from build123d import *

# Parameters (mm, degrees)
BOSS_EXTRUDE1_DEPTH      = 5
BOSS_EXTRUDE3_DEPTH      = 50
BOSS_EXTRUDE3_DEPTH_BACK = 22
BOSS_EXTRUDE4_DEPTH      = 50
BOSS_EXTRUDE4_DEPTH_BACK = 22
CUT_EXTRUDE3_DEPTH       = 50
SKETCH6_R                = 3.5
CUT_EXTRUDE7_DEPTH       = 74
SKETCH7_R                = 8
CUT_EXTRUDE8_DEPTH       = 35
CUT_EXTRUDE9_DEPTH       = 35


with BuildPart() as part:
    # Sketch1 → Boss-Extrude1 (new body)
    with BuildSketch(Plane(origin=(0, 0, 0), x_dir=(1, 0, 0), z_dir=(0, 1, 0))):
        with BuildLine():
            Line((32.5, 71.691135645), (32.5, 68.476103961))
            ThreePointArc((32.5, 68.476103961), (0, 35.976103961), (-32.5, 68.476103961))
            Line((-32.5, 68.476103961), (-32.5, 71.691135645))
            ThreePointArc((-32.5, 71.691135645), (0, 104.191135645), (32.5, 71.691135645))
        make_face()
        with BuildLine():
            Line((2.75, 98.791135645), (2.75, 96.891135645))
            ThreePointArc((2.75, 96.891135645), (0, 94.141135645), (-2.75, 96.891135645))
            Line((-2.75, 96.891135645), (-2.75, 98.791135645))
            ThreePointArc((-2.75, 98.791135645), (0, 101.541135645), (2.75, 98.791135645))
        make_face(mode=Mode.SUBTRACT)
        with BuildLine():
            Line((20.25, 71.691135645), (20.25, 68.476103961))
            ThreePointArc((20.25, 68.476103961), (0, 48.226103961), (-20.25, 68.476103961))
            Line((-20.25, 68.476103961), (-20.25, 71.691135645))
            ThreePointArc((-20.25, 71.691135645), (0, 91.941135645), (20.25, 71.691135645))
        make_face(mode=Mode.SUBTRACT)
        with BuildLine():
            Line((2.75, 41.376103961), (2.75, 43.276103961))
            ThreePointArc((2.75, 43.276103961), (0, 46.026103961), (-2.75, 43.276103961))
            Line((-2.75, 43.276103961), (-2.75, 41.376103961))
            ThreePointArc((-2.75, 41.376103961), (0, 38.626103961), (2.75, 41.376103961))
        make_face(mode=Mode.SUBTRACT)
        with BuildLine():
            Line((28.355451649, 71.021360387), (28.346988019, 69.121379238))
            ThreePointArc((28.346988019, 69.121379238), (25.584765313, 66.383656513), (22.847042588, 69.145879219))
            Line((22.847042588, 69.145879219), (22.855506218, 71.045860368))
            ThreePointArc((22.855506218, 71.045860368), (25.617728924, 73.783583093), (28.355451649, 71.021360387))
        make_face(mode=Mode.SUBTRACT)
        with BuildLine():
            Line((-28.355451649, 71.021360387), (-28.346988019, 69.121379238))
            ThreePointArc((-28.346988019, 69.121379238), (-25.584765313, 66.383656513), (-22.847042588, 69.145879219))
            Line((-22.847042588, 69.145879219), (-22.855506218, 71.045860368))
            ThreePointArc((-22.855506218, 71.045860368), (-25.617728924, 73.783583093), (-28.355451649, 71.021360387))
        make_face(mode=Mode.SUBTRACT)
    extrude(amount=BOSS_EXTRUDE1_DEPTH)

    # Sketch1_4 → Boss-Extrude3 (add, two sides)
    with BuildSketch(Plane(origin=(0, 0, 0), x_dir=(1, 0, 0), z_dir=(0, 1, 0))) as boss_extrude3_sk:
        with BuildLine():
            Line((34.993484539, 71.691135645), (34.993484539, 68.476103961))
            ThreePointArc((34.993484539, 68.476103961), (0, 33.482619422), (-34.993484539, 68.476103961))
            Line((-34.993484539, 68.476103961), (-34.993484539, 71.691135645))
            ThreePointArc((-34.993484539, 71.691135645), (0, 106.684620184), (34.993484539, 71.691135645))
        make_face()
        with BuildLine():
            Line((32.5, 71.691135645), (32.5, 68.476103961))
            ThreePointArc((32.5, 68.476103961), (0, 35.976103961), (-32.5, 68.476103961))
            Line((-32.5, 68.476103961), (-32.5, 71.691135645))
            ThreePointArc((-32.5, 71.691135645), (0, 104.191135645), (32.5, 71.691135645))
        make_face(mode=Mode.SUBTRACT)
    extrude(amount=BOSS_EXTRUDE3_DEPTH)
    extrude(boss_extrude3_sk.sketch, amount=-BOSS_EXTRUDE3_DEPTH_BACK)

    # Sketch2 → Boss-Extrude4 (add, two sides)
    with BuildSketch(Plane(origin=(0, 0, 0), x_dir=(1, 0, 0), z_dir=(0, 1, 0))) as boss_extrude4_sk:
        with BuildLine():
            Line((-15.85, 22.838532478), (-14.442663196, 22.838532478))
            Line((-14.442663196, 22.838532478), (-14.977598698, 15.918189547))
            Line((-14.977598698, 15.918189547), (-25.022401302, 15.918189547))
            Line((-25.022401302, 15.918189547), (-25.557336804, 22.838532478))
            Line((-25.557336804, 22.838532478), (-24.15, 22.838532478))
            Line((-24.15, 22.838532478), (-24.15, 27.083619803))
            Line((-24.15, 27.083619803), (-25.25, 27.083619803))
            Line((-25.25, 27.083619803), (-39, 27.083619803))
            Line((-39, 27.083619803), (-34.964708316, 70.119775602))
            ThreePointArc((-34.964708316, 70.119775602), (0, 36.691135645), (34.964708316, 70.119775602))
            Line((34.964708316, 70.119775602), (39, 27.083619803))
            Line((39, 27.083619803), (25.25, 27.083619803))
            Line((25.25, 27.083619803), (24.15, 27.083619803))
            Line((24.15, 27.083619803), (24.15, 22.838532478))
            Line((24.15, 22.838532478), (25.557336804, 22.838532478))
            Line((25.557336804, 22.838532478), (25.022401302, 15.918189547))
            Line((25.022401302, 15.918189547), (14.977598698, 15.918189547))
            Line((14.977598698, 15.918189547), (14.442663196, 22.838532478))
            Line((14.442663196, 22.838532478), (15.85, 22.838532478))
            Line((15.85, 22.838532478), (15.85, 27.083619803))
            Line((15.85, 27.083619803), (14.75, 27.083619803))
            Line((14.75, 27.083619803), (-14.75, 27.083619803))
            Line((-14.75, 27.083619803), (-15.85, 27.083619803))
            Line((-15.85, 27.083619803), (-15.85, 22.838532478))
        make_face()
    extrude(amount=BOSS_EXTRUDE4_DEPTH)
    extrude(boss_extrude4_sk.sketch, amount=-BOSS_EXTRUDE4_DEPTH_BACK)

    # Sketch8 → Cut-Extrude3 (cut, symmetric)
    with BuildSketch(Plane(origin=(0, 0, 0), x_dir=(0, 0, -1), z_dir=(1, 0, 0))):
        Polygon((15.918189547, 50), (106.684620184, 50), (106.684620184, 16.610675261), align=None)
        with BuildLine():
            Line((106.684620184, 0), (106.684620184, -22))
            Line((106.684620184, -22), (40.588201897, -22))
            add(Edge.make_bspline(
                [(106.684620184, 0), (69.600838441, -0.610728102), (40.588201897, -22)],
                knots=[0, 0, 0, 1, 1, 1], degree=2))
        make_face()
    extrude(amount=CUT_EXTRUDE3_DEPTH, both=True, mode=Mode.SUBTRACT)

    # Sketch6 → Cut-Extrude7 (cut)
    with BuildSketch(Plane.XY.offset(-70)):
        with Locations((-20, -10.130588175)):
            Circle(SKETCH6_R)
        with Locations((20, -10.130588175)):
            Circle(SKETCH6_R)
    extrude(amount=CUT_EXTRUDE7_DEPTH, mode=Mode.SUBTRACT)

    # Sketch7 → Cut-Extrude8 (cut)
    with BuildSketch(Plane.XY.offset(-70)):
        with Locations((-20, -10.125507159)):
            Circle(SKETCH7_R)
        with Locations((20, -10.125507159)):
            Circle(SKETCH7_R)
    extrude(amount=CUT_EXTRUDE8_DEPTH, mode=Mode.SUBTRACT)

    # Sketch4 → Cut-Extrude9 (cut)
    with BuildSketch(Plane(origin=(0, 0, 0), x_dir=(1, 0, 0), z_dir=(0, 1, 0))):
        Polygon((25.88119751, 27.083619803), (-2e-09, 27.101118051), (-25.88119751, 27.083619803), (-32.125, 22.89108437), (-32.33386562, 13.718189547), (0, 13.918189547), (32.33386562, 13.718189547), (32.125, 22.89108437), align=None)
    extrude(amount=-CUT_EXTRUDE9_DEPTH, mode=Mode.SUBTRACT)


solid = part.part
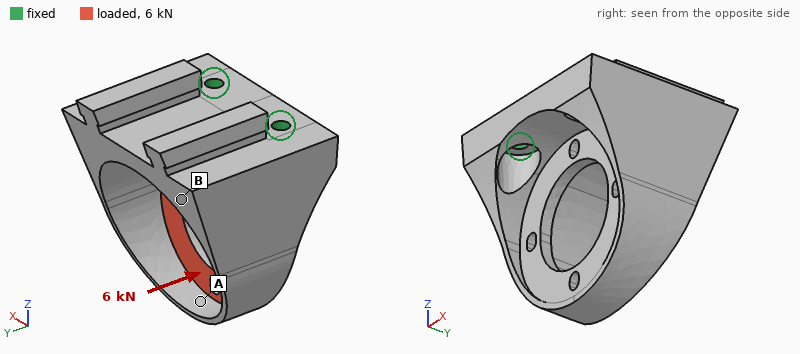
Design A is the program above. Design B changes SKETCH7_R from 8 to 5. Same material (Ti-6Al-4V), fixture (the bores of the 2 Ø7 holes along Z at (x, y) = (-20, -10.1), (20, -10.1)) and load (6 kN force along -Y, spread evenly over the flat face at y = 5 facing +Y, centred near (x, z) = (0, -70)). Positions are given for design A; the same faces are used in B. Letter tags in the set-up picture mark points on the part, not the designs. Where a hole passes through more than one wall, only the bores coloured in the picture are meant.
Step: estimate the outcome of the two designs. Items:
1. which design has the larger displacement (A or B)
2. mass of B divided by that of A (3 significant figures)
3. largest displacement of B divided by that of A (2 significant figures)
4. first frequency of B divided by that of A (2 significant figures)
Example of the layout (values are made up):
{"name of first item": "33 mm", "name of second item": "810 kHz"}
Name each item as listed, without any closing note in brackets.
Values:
{"which design has the larger displacement": "A", "mass of B divided by that of A": "1.02", "largest displacement of B divided by that of A": "0.90", "first frequency of B divided by that of A": "1.1"}
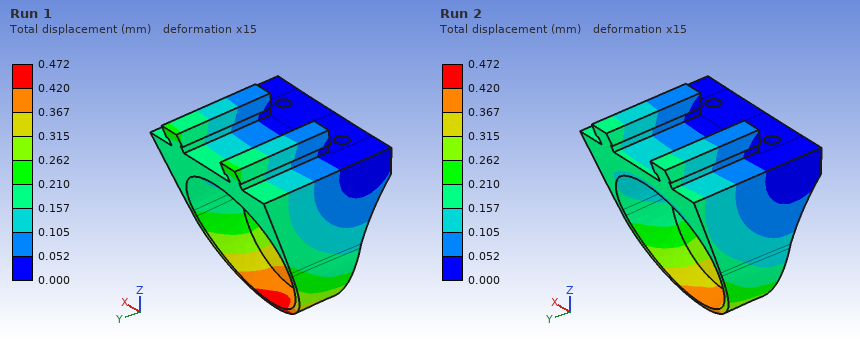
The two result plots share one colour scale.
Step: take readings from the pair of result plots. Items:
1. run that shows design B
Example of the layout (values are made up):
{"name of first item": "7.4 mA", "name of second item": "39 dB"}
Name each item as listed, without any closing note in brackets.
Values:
{"run that shows design B": "Run 2"}
